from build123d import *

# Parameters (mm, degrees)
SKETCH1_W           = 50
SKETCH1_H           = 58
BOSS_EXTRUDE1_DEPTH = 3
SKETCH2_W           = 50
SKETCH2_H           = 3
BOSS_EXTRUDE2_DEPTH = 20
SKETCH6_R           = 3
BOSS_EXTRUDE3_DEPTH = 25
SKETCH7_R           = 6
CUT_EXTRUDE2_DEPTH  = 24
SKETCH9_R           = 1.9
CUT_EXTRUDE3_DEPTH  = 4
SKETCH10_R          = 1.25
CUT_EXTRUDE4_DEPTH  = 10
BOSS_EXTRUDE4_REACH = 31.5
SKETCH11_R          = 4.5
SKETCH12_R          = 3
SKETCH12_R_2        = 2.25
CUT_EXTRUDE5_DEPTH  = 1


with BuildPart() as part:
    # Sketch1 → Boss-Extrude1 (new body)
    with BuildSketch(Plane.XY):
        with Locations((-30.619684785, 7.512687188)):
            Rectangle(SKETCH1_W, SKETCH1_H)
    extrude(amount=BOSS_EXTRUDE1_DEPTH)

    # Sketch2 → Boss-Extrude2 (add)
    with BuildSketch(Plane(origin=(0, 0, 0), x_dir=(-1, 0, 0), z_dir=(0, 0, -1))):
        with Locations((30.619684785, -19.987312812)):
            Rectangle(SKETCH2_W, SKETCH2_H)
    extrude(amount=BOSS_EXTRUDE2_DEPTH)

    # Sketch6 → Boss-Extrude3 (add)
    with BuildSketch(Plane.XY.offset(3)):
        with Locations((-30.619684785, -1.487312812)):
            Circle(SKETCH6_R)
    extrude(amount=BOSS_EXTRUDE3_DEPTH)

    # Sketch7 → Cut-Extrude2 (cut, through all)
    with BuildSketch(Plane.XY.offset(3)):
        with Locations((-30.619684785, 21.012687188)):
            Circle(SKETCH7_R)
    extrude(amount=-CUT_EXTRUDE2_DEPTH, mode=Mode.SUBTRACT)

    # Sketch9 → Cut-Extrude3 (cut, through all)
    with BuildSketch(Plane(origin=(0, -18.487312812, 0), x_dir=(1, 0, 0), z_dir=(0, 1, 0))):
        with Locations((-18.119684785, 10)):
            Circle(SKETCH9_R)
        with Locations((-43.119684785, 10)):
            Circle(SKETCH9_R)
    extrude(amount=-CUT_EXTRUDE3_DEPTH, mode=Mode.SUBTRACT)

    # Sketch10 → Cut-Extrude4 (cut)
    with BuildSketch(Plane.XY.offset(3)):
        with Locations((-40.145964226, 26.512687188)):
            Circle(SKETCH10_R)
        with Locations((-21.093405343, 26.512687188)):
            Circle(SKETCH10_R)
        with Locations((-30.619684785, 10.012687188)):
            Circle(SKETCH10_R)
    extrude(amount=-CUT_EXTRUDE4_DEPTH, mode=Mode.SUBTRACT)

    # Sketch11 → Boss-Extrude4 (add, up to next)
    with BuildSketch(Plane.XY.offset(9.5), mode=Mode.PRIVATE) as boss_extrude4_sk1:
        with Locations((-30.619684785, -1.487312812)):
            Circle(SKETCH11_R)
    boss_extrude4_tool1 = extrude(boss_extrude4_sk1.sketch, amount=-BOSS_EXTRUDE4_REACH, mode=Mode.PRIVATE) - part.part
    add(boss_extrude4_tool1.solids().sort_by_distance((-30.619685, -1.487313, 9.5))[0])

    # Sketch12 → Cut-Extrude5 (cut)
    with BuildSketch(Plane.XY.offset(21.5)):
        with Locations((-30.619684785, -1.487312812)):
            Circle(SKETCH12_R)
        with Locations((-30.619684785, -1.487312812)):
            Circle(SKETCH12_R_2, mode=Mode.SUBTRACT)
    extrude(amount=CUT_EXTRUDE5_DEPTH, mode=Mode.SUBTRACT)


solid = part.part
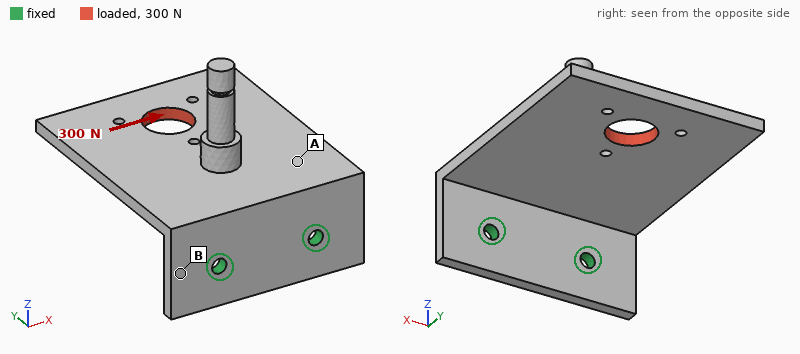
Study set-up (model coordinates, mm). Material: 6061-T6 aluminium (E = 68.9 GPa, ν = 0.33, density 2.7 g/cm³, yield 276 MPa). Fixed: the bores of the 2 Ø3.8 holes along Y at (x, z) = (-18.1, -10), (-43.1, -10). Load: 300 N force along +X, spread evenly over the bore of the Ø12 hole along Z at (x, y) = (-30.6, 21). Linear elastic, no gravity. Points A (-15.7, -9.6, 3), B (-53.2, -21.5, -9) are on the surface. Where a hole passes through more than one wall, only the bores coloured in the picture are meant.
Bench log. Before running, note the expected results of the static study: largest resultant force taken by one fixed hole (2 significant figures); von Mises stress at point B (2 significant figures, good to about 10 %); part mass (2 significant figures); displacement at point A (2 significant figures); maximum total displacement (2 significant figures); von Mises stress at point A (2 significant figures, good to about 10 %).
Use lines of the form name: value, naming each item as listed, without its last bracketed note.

largest resultant force taken by one fixed hole: 460 N
von Mises stress at point B: 37 MPa
part mass: 33 g
displacement at point A: 0.056 mm
maximum total displacement: 0.19 mm
von Mises stress at point A: 15 MPa
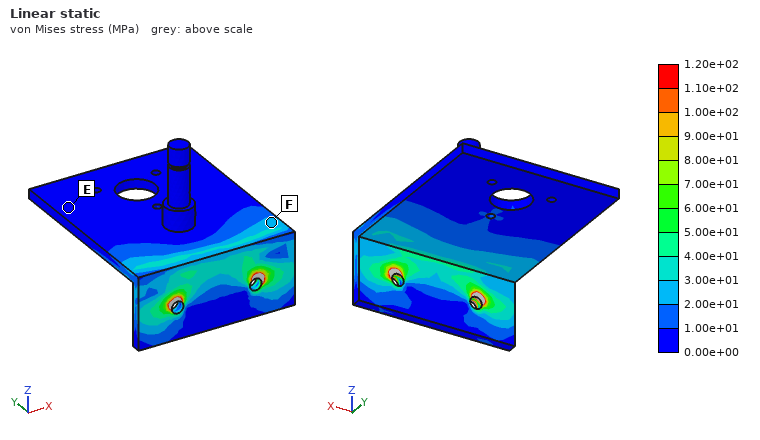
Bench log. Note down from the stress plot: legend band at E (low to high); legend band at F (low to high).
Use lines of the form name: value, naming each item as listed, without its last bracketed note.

legend band at E: 0.00e+00 to 1.00e+01 MPa
legend band at F: 2.00e+01 to 3.00e+01 MPa
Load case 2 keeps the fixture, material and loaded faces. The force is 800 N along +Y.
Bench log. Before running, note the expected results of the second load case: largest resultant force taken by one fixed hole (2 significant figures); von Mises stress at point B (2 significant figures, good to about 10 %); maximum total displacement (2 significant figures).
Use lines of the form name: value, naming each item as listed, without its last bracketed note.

largest resultant force taken by one fixed hole: 400 N
von Mises stress at point B: 43 MPa
maximum total displacement: 0.41 mm
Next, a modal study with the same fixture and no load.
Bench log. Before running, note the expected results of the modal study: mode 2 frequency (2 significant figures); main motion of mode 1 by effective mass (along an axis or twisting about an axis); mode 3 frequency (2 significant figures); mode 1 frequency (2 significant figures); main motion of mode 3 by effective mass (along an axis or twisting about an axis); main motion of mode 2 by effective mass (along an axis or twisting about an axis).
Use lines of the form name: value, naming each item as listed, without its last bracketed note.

mode 2 frequency: 1700 Hz
main motion of mode 1 by effective mass: along Z
mode 3 frequency: 2300 Hz
mode 1 frequency: 600 Hz
main motion of mode 3 by effective mass: along X
main motion of mode 2 by effective mass: along X
